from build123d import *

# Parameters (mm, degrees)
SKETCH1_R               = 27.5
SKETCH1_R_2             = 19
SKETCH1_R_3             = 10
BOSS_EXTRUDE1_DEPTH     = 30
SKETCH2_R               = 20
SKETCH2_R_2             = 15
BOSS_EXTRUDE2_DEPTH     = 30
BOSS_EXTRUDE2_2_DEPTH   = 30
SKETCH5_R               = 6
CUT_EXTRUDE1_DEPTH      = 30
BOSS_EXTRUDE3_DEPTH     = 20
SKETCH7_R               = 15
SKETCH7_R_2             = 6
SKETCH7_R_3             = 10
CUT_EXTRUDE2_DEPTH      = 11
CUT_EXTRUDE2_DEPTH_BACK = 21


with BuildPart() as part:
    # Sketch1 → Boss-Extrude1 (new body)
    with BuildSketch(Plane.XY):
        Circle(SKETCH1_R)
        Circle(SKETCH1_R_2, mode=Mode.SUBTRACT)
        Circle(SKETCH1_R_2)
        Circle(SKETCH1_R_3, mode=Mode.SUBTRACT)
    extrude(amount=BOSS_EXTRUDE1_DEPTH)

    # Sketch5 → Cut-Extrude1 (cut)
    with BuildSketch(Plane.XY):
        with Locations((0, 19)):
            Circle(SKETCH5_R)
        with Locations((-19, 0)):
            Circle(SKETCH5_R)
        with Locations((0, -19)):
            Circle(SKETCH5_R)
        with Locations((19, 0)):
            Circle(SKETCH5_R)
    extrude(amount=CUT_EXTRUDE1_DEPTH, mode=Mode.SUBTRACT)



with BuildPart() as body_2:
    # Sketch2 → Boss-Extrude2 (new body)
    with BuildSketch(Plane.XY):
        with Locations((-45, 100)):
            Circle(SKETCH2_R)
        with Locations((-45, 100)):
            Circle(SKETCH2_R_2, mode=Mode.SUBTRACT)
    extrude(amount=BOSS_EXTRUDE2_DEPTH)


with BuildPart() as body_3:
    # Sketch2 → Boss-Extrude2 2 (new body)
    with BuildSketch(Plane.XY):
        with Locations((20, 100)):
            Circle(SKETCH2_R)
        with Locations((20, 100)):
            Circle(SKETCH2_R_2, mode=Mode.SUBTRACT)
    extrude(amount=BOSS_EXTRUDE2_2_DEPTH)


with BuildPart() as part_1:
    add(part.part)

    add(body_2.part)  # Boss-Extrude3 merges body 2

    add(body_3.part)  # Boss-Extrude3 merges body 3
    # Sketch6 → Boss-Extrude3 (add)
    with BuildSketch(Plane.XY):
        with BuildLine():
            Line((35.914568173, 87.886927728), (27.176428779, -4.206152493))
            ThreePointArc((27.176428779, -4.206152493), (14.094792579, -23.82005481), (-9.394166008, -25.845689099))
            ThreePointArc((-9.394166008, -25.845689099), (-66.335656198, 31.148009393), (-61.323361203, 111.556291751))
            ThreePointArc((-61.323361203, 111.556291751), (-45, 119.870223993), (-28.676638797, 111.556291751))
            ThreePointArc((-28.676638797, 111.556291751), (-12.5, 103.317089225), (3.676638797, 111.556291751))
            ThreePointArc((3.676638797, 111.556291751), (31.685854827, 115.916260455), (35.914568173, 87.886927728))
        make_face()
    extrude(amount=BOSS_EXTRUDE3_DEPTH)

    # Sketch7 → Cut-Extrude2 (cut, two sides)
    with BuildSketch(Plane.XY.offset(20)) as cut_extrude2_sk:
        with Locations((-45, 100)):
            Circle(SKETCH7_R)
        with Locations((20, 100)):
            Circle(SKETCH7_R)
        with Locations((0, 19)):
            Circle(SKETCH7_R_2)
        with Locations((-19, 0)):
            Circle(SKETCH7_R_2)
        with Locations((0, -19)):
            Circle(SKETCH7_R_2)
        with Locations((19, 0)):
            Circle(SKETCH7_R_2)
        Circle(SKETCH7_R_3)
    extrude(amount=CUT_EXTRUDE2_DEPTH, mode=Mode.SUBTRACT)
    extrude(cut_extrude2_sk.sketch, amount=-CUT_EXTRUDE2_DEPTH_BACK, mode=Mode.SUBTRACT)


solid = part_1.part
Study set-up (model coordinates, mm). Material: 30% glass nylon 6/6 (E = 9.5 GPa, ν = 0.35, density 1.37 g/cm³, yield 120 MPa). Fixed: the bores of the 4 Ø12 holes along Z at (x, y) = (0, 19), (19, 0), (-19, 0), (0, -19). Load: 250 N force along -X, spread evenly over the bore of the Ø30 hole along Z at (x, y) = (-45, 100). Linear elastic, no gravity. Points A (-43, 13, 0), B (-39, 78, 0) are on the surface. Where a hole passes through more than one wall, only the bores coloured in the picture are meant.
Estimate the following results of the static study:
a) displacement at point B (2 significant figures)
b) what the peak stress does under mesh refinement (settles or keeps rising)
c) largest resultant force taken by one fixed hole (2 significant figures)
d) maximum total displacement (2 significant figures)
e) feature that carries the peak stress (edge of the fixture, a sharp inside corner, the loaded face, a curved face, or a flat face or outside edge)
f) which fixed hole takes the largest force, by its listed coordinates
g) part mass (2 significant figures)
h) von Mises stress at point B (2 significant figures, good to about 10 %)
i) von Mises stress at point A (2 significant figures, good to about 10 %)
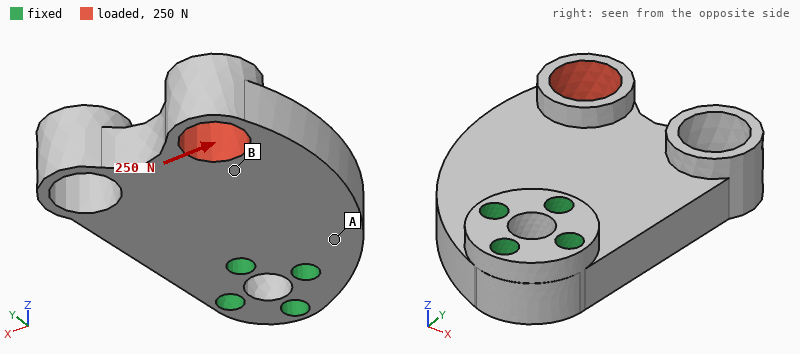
11 µm
keeps rising
440 N
29 µm
a sharp inside corner
(0, 19)
330 g
0.27 MPa
0.62 MPa
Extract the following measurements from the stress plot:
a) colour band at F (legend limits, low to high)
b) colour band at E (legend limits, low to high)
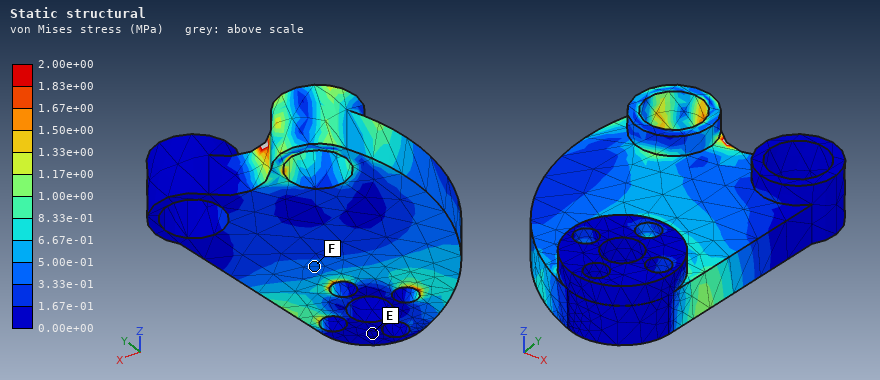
3.33e-01 to 5.00e-01 MPa
0.00e+00 to 1.67e-01 MPa
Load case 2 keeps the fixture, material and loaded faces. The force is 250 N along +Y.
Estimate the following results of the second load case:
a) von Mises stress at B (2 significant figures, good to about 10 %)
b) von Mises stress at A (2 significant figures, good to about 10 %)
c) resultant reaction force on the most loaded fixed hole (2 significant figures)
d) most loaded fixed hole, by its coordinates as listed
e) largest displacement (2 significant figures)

0.15 MPa
0.24 MPa
260 N
(-19, 0)
20 µm
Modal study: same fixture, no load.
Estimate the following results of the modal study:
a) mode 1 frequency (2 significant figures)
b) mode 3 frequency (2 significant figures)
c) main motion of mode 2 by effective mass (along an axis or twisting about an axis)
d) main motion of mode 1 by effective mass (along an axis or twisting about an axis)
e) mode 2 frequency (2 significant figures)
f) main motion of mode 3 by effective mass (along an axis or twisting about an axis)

880 Hz
1900 Hz
twisting about Y
along Z
1500 Hz
along X
